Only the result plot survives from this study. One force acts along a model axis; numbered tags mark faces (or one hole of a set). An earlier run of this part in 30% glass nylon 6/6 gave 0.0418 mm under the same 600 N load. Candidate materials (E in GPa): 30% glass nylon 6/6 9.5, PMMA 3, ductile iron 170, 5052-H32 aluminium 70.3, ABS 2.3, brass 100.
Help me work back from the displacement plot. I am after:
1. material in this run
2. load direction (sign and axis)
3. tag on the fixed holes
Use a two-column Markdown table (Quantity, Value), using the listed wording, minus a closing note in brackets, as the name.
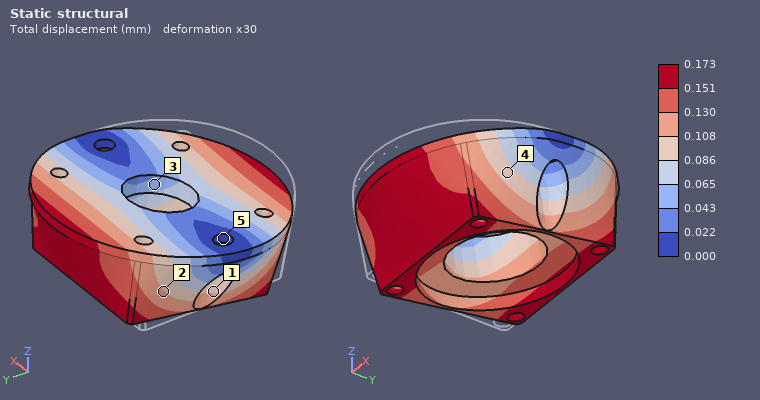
| Quantity | Value |
|---|---|
| material in this run | ABS |
| load direction | +Y |
| tag on the fixed holes | 5 |
